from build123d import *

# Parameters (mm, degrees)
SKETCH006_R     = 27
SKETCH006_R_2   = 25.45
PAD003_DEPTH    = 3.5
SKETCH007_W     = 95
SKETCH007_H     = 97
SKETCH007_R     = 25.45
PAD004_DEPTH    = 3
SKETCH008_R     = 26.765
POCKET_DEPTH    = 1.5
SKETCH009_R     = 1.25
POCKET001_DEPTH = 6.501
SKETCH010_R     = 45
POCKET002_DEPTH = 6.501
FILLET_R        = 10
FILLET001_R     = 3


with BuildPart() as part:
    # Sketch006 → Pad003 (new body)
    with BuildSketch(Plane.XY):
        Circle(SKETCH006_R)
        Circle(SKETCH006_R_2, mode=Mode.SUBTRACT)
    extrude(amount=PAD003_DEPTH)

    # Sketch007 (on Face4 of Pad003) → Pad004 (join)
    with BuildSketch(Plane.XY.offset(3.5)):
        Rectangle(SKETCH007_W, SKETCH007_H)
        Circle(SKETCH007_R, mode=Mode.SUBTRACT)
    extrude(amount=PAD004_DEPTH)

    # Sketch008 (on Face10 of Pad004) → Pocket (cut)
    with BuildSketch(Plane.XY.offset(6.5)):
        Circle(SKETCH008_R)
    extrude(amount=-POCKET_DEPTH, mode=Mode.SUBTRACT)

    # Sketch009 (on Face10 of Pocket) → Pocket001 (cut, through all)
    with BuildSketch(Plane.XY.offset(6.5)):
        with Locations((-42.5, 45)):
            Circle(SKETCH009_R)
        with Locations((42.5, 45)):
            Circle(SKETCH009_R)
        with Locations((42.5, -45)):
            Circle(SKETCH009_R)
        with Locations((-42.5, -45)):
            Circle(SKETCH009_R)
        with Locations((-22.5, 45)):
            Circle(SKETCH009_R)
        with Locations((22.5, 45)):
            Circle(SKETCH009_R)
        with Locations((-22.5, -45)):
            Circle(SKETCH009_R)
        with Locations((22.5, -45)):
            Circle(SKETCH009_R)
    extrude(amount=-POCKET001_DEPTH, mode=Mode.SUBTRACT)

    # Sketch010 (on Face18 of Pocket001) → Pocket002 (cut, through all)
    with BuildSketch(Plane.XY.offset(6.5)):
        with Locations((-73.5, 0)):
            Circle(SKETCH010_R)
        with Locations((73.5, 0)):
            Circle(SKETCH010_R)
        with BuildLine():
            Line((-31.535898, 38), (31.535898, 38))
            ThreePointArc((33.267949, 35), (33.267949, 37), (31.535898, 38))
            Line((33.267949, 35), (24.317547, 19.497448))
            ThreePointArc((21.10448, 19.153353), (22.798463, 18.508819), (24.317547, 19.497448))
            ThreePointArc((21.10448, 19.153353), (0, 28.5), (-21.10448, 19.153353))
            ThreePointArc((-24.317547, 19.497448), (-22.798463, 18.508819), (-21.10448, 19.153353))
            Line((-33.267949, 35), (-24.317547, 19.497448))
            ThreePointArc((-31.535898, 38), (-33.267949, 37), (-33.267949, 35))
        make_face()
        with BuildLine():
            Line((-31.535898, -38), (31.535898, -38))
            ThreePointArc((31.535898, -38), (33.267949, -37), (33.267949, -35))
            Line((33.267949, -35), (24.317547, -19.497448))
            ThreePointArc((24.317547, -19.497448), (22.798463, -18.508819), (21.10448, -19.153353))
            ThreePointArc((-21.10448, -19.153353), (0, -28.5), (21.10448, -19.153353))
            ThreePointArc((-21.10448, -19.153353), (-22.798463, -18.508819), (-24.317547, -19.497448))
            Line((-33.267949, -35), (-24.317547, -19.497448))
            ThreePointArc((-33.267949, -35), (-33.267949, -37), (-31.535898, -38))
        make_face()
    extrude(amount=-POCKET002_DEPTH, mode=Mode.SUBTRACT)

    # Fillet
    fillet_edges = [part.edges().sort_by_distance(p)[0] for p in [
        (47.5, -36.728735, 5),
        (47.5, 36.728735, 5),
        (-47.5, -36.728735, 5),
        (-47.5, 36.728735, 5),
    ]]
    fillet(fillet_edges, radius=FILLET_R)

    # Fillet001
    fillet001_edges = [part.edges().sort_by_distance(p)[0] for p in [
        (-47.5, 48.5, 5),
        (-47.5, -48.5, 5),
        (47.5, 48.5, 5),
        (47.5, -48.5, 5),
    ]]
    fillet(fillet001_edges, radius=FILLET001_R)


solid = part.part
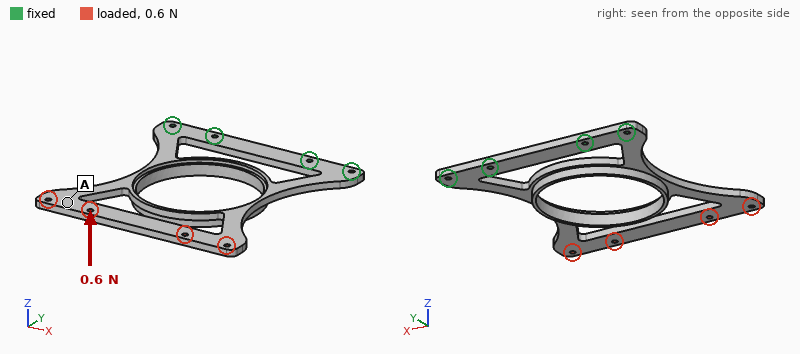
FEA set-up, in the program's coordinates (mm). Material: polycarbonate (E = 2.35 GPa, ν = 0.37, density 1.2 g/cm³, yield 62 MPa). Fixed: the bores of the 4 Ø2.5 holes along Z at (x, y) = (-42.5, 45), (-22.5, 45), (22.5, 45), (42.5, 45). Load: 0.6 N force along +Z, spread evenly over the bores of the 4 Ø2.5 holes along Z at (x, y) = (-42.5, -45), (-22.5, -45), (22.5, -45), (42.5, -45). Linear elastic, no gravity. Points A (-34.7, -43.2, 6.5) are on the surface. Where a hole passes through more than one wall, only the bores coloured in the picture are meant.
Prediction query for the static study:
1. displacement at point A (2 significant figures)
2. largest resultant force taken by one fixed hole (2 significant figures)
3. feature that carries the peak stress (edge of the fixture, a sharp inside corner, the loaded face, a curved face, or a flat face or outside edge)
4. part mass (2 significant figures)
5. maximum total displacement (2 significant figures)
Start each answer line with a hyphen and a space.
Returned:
- 1.4 mm
- 0.36 N
- a curved face
- 13 g
- 1.6 mm
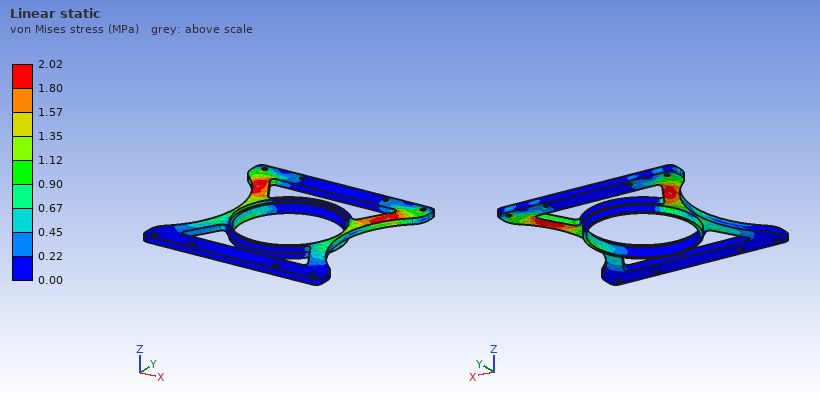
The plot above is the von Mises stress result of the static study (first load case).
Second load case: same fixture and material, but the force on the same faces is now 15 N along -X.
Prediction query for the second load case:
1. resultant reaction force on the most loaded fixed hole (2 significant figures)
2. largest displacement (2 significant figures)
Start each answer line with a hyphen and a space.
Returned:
- 19 N
- 1.6 mm
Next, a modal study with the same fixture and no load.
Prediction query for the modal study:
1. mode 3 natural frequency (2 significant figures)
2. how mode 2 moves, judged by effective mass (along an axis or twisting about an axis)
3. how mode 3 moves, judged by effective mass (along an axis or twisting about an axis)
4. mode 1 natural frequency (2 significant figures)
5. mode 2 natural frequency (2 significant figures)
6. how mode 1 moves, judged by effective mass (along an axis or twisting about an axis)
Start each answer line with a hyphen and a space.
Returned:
- 230 Hz
- twisting about Y
- along X
- 47 Hz
- 110 Hz
- along Z
